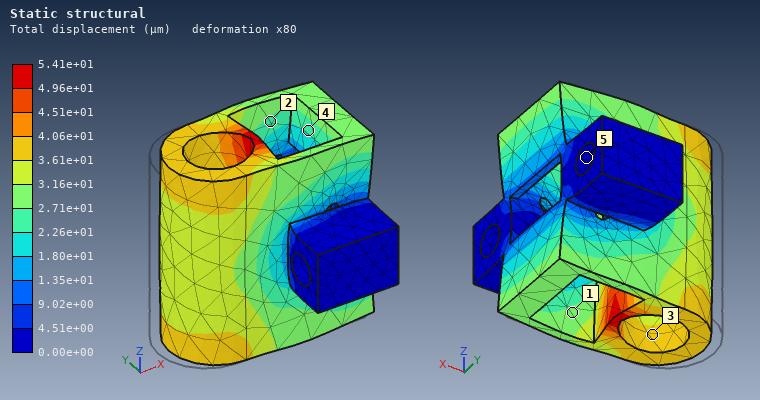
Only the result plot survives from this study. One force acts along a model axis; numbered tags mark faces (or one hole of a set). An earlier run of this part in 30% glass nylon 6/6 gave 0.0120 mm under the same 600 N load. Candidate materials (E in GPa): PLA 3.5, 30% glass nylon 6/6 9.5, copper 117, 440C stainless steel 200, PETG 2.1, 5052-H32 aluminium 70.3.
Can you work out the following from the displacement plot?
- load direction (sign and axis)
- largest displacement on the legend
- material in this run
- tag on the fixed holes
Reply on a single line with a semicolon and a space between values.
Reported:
+X; 5.41e+01 µm; PETG; 5
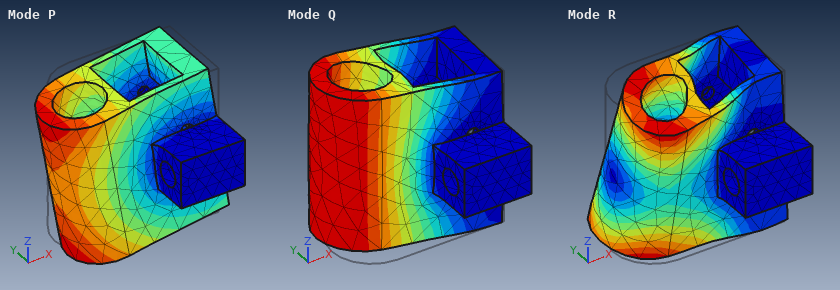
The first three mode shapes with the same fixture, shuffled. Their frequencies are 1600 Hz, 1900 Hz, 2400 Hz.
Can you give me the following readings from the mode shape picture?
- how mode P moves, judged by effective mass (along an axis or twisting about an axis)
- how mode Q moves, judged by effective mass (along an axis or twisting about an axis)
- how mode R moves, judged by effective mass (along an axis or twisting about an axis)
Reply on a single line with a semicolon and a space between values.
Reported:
along Z; along Y; twisting about X
